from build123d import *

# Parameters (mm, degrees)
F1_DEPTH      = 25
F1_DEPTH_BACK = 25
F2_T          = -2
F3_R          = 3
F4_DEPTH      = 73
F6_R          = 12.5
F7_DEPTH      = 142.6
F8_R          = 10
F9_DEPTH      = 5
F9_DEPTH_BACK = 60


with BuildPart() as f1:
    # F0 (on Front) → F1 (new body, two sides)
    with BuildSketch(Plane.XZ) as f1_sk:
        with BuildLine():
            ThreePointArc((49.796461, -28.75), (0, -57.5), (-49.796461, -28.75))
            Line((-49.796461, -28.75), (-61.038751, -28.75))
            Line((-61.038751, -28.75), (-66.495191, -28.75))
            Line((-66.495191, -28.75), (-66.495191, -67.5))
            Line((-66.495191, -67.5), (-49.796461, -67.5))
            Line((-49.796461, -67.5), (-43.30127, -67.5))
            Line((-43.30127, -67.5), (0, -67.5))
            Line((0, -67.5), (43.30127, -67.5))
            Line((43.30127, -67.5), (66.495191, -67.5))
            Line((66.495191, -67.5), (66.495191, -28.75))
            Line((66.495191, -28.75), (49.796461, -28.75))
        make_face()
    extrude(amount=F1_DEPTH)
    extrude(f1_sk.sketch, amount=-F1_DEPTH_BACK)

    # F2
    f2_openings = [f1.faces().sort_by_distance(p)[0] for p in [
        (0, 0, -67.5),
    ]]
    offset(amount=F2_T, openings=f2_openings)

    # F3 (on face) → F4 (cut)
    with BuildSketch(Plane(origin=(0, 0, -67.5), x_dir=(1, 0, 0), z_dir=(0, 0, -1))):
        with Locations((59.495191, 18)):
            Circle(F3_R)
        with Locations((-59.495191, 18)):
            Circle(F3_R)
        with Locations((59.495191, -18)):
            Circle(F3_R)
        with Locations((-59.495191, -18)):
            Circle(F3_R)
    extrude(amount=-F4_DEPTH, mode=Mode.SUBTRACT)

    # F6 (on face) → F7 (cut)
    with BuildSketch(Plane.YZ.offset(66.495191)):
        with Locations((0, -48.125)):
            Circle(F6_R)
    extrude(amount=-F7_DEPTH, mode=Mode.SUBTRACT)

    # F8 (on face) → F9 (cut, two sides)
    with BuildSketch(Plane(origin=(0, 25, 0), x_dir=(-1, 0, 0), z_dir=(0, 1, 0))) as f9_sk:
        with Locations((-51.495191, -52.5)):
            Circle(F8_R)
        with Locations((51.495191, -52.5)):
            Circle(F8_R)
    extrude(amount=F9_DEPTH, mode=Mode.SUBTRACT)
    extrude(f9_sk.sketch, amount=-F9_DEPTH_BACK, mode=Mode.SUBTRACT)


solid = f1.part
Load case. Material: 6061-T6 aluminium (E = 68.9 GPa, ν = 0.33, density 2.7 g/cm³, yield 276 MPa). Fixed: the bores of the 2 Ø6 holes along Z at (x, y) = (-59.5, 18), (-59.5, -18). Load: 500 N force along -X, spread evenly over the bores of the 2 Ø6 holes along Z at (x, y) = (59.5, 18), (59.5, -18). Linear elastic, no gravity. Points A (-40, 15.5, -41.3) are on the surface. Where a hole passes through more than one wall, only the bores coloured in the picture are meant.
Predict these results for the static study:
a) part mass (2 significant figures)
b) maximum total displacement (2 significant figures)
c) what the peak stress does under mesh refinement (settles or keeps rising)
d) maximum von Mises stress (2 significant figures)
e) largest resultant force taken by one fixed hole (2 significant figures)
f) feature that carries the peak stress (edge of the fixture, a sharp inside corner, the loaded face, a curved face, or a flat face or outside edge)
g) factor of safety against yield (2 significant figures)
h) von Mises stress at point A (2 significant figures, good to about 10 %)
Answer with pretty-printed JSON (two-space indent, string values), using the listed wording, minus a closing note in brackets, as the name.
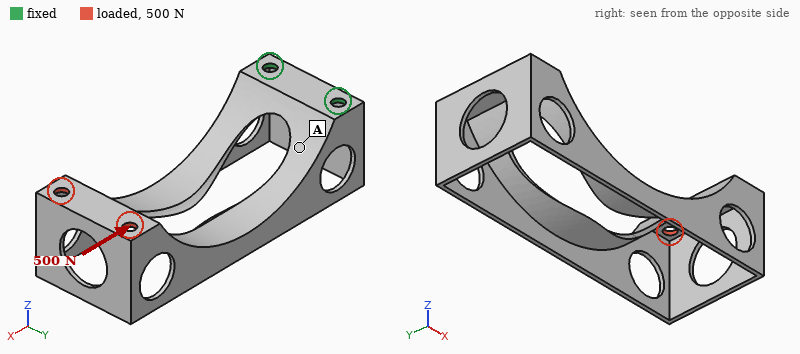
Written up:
{
  "part mass": "66 g",
  "maximum total displacement": "1.5 mm",
  "what the peak stress does under mesh refinement": "settles",
  "maximum von Mises stress": "180 MPa",
  "largest resultant force taken by one fixed hole": "250 N",
  "feature that carries the peak stress": "a flat face or outside edge",
  "factor of safety against yield": "1.5",
  "von Mises stress at point A": "24 MPa"
}
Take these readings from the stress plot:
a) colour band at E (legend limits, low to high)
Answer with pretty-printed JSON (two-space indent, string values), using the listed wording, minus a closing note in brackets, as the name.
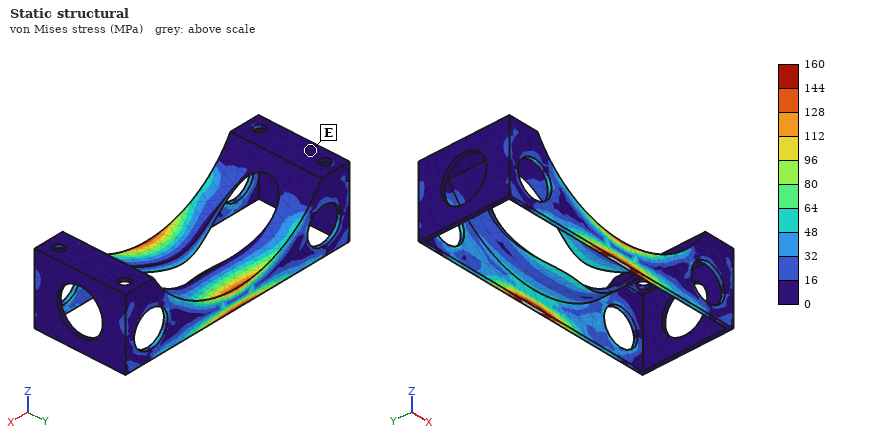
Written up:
{
  "colour band at E": "0 to 16 MPa"
}
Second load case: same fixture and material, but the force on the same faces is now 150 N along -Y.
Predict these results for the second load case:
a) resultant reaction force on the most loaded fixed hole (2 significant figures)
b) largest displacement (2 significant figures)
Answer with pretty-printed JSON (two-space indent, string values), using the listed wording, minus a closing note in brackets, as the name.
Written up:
{
  "resultant reaction force on the most loaded fixed hole": "380 N",
  "largest displacement": "1.7 mm"
}
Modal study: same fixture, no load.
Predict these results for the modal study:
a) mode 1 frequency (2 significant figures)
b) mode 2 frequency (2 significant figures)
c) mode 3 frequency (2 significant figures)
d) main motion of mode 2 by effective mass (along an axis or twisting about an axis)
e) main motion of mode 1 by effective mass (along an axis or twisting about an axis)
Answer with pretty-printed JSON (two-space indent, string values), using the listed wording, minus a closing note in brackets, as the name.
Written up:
{
  "mode 1 frequency": "290 Hz",
  "mode 2 frequency": "360 Hz",
  "mode 3 frequency": "530 Hz",
  "main motion of mode 2 by effective mass": "along Y",
  "main motion of mode 1 by effective mass": "along Z"
}
